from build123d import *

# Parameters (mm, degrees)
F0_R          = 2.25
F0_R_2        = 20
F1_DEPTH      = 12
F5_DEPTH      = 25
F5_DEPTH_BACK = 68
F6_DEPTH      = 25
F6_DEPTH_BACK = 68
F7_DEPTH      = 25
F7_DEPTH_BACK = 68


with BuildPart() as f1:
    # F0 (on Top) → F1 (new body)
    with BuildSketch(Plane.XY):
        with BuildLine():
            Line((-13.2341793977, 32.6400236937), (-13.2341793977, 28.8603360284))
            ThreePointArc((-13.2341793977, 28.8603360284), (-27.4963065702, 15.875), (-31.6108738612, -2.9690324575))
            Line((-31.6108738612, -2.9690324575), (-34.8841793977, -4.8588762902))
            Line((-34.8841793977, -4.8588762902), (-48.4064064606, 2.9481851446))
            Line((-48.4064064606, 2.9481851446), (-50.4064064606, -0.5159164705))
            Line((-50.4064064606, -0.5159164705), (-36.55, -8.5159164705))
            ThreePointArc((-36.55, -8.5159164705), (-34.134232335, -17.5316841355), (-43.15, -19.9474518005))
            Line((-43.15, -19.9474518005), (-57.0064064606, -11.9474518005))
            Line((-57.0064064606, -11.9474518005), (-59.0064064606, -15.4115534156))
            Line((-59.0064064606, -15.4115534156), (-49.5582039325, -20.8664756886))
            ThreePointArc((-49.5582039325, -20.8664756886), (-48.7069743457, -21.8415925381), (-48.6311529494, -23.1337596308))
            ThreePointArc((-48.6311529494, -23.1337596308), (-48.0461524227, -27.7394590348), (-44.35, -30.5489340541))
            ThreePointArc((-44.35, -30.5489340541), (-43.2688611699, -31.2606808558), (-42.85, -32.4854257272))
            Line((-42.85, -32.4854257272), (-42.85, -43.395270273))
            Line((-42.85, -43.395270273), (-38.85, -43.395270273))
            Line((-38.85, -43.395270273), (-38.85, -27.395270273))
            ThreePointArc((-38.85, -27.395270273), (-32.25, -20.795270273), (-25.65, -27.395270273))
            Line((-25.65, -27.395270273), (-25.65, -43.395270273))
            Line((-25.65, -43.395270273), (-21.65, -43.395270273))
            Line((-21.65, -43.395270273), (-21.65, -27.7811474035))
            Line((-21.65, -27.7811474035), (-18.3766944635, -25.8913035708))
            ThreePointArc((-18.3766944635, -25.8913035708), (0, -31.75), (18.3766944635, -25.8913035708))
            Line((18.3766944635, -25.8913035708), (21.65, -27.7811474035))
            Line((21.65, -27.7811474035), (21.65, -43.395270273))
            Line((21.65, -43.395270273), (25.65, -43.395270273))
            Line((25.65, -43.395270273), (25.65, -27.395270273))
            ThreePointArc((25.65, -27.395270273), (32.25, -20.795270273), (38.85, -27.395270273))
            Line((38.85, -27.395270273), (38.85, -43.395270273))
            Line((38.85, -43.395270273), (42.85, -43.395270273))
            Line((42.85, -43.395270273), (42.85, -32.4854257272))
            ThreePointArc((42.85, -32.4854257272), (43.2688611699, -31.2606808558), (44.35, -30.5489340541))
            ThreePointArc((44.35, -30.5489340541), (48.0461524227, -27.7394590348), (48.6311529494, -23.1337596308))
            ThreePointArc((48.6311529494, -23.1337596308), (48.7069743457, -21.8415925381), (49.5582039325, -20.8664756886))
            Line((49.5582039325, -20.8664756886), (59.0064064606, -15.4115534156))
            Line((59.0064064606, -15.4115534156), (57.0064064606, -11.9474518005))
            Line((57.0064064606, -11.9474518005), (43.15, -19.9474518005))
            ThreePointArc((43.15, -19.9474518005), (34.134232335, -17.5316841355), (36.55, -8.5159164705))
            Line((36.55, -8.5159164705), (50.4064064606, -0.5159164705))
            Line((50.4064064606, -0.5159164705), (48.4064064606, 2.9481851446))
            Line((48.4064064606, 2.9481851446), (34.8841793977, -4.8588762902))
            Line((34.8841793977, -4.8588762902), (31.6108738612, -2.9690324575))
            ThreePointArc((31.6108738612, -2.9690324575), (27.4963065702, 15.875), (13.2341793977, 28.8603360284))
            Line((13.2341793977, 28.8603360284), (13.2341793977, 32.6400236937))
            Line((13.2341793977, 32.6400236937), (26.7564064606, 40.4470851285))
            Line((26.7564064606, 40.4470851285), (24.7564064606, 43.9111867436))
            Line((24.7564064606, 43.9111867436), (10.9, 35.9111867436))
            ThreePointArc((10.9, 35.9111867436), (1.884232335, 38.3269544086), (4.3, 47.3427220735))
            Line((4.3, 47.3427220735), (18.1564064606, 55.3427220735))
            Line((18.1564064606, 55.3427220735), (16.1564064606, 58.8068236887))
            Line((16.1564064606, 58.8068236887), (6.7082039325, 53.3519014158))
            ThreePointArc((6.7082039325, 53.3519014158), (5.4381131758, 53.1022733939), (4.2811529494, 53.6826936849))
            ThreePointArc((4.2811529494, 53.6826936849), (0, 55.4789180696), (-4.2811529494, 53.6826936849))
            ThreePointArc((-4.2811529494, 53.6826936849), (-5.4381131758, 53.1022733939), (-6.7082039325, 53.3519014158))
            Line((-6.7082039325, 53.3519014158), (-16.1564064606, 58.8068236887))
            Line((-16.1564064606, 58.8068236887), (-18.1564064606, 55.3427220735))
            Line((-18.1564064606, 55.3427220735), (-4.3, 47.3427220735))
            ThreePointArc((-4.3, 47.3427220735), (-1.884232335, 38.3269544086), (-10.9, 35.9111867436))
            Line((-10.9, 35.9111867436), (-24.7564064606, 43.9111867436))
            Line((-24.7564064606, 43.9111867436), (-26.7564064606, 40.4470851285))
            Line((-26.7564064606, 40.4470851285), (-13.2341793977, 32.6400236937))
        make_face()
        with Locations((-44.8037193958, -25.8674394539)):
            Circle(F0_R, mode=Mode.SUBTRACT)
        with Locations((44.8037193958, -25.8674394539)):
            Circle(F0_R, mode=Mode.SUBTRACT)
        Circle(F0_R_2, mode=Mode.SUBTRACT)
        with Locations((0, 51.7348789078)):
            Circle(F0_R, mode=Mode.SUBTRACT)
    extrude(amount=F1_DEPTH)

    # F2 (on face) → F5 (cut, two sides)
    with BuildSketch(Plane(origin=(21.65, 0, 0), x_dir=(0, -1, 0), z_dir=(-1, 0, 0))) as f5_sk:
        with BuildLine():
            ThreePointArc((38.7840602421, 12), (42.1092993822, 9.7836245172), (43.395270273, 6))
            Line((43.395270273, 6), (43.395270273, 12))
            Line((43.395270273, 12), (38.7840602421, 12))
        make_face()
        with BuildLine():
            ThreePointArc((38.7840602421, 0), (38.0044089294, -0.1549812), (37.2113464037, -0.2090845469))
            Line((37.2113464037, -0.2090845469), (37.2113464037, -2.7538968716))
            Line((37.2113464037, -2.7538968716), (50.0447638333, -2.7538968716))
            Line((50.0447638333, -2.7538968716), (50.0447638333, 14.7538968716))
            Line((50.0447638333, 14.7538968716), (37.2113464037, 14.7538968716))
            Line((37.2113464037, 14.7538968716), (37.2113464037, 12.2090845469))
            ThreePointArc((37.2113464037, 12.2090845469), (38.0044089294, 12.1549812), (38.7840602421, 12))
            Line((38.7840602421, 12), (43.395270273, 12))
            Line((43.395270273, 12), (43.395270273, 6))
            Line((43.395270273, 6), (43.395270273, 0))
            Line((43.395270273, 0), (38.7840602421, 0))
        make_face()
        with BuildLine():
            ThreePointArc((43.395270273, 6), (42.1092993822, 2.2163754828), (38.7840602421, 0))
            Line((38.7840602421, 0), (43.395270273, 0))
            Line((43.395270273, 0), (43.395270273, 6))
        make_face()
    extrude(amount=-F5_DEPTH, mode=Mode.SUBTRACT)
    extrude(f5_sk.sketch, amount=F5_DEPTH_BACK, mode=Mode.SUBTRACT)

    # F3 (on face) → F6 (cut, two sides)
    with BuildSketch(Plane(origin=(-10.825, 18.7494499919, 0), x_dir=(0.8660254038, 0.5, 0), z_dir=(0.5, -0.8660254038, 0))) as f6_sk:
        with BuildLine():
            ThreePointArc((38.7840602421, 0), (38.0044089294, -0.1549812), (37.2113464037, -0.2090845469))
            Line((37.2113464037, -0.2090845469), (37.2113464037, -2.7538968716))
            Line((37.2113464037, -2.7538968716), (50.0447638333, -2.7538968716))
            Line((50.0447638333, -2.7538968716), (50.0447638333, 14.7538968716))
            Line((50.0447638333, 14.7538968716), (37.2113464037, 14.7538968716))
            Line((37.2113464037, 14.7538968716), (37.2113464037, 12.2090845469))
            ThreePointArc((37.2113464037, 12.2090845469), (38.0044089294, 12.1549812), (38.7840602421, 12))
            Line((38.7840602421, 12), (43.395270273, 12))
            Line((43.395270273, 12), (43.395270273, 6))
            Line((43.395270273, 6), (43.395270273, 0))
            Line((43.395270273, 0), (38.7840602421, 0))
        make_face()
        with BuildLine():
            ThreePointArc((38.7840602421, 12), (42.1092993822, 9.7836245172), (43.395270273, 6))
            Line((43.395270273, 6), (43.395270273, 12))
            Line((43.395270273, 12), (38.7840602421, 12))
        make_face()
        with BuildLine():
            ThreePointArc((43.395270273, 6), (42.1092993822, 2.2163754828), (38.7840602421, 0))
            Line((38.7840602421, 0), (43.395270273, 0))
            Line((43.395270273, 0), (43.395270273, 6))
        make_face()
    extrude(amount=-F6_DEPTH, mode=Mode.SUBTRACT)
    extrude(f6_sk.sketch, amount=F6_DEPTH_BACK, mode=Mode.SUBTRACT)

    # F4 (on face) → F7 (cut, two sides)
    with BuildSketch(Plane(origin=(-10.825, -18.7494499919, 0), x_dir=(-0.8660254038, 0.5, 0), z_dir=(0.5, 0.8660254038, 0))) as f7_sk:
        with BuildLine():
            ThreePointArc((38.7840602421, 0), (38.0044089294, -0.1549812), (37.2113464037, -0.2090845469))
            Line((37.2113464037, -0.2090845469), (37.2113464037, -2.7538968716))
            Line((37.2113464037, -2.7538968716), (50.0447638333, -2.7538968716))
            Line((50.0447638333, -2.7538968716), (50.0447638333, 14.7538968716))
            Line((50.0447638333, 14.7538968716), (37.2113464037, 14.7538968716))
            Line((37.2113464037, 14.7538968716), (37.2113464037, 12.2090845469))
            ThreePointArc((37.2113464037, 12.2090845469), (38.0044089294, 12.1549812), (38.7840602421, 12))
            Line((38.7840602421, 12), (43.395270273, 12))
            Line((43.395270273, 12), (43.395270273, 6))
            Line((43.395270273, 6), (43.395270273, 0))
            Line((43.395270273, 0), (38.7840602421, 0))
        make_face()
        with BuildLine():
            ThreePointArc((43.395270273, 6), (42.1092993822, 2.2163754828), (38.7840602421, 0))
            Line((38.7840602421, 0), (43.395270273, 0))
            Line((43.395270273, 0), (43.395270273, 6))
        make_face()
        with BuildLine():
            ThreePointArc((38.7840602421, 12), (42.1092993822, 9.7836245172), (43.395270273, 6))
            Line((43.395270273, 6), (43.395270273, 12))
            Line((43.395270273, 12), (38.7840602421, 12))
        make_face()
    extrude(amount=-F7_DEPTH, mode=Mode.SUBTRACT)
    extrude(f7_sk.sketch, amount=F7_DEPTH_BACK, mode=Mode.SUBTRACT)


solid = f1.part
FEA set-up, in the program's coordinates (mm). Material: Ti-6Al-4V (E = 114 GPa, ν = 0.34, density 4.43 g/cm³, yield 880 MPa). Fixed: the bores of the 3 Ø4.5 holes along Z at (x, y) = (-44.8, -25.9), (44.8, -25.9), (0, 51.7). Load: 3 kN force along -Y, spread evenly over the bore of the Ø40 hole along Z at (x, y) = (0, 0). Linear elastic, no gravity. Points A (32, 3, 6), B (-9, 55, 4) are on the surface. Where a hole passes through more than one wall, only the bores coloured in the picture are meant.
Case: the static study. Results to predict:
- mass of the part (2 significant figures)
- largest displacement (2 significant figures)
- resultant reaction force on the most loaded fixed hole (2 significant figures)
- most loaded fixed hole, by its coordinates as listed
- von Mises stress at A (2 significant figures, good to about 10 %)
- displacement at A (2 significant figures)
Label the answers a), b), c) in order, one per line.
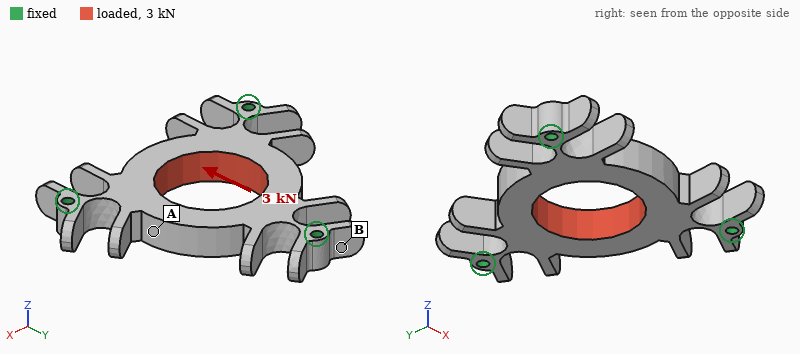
a) 170 g
b) 21 µm
c) 1.6 kN
d) (0, 51.7)
e) 17 MPa
f) 15 µm
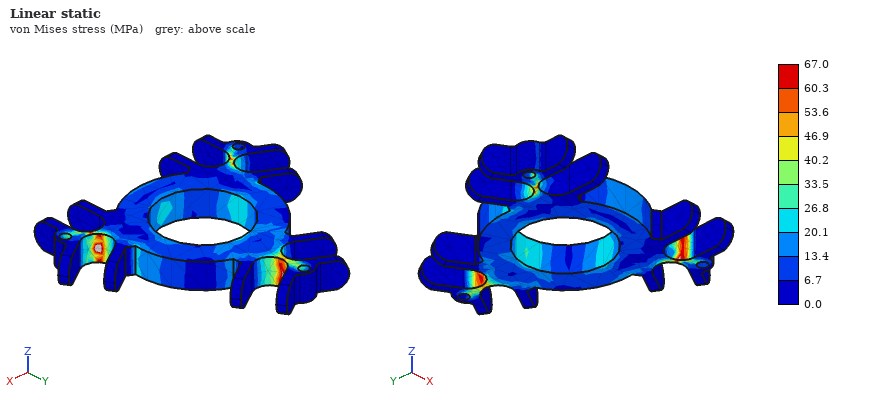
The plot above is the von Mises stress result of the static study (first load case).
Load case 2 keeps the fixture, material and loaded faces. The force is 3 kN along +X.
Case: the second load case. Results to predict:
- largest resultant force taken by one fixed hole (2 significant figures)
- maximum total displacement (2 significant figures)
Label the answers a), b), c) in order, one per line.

a) 1.4 kN
b) 20 µm
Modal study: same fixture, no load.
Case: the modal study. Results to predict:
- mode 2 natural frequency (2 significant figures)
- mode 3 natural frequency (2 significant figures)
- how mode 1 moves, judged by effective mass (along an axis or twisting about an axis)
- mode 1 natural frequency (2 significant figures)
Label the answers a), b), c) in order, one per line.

a) 4400 Hz
b) 4400 Hz
c) along Z
d) 4200 Hz
